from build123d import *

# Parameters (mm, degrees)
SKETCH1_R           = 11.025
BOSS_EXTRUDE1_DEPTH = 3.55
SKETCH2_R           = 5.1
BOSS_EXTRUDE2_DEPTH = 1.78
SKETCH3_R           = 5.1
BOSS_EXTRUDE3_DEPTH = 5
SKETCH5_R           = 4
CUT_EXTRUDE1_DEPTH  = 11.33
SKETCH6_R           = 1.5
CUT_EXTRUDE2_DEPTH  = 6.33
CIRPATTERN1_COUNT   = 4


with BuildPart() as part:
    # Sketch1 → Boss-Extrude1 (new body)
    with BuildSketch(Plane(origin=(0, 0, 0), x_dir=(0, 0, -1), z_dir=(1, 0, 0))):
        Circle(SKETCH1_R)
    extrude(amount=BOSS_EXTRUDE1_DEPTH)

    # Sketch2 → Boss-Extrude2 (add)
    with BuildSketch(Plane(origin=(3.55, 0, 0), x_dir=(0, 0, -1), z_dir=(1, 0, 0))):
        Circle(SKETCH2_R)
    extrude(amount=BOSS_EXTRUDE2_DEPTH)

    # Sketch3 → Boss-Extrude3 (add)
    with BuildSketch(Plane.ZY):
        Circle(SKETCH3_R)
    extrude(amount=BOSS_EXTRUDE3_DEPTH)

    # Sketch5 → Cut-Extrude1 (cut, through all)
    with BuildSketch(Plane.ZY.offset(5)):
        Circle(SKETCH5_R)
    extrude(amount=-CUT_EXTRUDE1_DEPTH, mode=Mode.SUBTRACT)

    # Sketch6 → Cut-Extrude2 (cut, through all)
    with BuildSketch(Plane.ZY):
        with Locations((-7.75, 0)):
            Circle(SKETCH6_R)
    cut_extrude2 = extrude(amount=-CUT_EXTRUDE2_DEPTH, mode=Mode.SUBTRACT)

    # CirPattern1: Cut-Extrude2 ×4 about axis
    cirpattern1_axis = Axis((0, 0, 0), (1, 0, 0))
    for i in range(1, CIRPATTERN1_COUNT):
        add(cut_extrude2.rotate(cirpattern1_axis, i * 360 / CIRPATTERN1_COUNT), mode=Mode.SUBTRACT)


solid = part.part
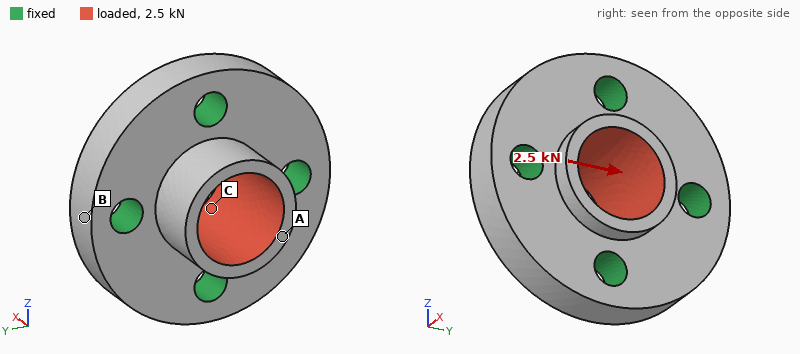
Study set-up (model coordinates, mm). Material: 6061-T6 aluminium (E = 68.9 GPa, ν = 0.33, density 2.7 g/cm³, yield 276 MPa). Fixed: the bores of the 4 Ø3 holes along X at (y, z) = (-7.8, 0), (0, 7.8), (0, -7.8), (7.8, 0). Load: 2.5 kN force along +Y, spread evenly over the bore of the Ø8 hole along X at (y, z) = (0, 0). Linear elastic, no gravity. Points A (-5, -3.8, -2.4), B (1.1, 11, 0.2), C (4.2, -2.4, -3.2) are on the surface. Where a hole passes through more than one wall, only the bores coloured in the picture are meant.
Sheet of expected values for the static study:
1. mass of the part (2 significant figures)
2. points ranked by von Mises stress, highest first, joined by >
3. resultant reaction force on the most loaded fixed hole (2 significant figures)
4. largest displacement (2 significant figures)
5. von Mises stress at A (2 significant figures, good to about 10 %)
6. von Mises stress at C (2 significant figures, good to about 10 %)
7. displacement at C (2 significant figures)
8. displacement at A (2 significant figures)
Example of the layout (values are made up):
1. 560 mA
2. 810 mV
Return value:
1. 3.5 g
2. A > C > B
3. 740 N
4. 15 µm
5. 51 MPa
6. 31 MPa
7. 2.8 µm
8. 14 µm
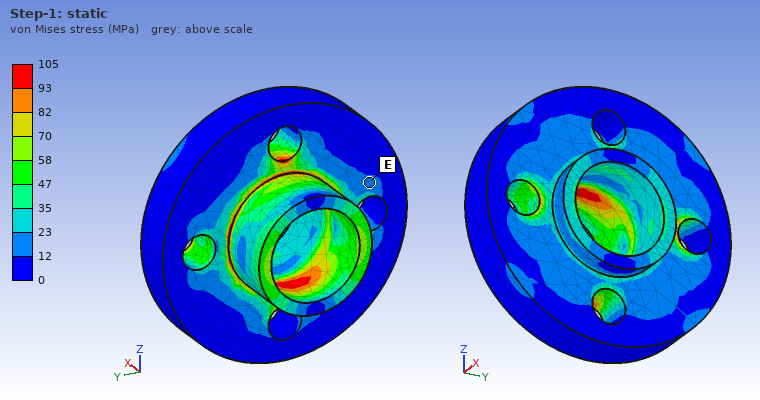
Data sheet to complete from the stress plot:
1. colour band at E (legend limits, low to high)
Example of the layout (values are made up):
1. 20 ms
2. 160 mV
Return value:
1. 12 to 23 MPa
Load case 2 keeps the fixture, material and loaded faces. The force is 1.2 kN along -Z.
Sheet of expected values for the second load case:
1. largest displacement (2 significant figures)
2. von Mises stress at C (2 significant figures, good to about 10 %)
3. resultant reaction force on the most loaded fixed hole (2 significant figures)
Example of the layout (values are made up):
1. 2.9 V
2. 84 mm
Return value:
1. 7.3 µm
2. 12 MPa
3. 360 N
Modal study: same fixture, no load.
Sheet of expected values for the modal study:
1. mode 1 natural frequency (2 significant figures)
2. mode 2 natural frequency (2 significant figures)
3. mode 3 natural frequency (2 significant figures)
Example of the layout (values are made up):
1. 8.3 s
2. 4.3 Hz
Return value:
1. 68 kHz
2. 73 kHz
3. 80 kHz
